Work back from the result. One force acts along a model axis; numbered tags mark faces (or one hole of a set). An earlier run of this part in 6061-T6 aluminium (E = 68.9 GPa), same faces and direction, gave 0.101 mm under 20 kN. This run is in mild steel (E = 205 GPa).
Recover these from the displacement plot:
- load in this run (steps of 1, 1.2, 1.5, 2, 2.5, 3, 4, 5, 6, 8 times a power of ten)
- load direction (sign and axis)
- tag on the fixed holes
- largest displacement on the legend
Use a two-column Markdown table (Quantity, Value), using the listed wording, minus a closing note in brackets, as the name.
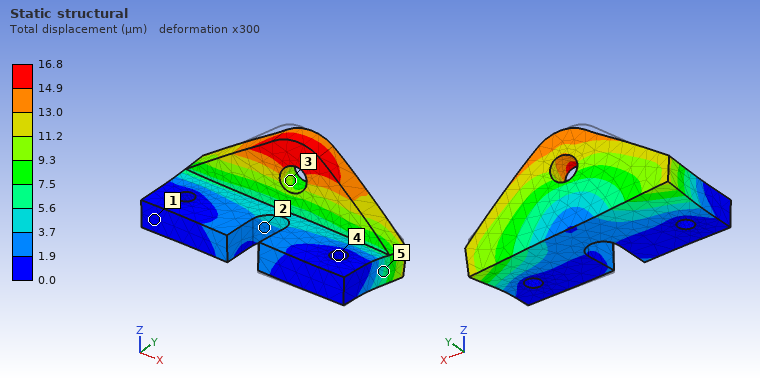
| Quantity | Value |
|---|---|
| load in this run | 10 kN |
| load direction | +X |
| tag on the fixed holes | 4 |
| largest displacement on the legend | 16.8 µm |
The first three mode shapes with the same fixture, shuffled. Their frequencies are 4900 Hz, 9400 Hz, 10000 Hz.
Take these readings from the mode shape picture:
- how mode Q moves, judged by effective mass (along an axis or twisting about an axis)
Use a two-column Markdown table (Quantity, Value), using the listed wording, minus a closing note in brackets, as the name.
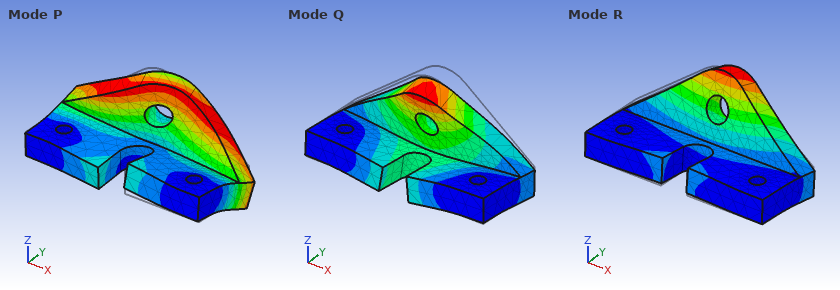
| Quantity | Value |
|---|---|
| how mode Q moves, judged by effective mass | along Z |
